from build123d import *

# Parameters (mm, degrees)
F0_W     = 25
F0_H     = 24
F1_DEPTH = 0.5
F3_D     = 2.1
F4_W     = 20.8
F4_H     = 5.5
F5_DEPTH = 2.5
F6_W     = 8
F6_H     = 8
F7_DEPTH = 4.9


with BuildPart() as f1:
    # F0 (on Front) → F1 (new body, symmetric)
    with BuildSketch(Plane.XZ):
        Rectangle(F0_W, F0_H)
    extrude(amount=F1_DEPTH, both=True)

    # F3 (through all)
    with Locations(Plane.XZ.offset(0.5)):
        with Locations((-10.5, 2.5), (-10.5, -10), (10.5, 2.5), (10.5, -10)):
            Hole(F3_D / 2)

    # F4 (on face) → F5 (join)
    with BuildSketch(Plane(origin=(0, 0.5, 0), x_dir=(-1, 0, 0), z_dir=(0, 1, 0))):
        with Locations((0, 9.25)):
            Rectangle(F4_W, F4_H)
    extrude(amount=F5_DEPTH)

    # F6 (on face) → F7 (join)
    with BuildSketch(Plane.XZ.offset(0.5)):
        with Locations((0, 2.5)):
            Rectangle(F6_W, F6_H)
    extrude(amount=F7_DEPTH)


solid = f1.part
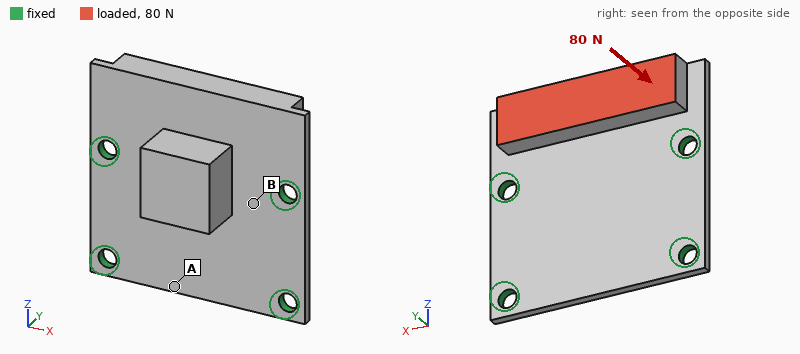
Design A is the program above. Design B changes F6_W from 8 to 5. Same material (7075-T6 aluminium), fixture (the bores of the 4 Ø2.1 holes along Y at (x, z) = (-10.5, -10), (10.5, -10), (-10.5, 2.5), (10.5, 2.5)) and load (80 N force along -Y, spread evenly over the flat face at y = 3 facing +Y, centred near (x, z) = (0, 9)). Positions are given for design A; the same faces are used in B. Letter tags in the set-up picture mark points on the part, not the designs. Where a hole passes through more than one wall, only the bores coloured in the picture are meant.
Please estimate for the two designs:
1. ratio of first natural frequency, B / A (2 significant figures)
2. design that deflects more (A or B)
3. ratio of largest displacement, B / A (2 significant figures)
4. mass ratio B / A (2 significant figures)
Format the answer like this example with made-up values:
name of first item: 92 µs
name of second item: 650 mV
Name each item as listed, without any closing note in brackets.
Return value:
ratio of first natural frequency, B / A: 0.97
design that deflects more: B
ratio of largest displacement, B / A: 1.1
mass ratio B / A: 0.90
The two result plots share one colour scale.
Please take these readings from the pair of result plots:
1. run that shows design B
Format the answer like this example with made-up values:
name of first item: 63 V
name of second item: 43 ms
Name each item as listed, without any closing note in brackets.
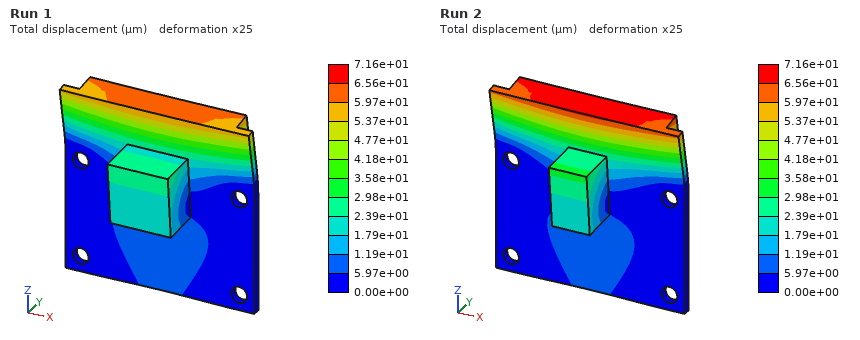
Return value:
run that shows design B: Run 2
